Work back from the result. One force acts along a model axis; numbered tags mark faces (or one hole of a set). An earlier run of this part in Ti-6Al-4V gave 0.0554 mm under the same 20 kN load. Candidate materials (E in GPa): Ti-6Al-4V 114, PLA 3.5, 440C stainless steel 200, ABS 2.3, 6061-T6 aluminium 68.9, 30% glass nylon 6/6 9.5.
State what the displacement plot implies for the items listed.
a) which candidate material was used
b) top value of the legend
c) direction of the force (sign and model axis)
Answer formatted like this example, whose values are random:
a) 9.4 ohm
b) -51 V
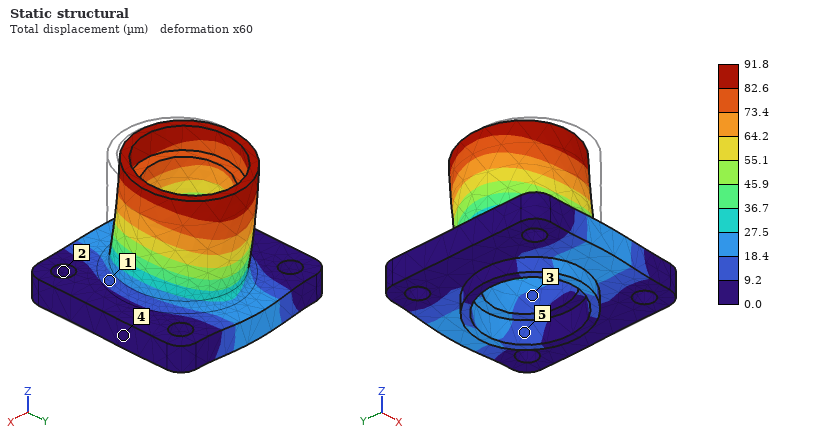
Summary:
a) 6061-T6 aluminium
b) 91.8 µm
c) +Y
